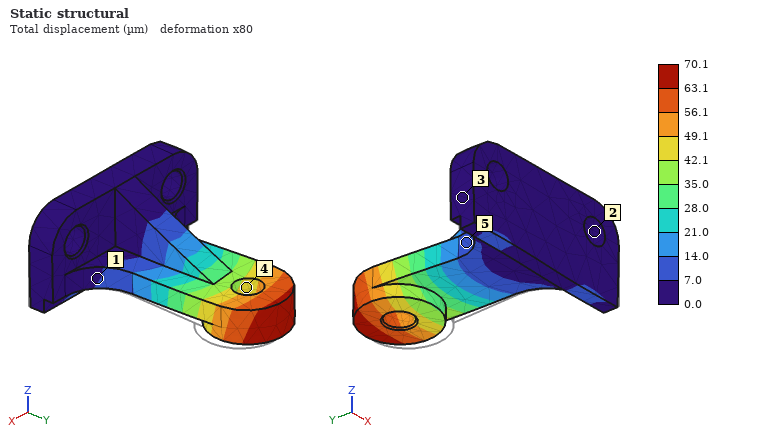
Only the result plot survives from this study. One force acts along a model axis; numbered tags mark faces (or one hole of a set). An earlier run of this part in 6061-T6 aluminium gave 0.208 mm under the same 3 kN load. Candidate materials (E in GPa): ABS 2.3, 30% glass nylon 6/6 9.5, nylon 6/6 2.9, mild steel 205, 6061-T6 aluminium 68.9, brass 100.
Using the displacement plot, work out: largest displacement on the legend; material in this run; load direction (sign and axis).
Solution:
70.1 µm
mild steel
-X
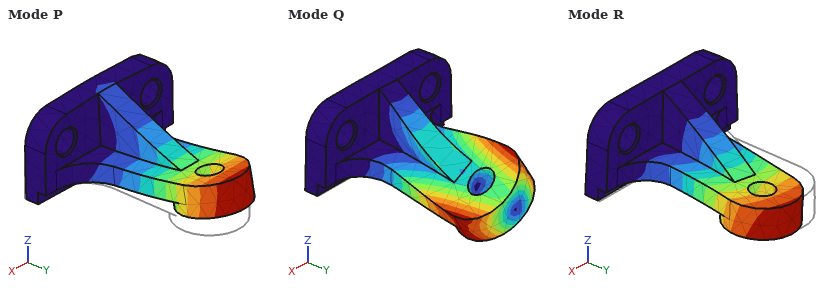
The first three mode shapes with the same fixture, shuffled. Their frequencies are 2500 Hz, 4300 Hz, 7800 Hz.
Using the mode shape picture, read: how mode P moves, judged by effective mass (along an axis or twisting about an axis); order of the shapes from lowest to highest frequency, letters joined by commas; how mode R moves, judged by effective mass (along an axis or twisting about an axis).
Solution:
along Z
P, R, Q
along X
